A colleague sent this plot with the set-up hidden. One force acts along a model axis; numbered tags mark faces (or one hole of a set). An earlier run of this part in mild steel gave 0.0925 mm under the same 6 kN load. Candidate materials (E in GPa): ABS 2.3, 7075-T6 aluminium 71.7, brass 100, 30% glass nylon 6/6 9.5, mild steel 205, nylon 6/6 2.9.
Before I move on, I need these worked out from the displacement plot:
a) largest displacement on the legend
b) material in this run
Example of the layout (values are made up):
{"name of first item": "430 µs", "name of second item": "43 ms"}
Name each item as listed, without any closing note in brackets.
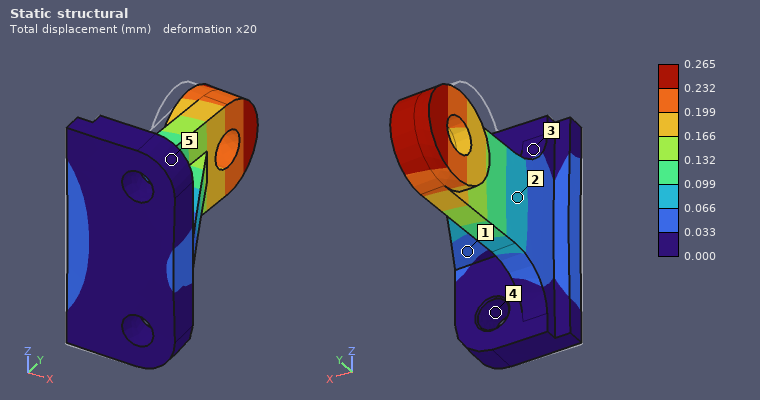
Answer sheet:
{"largest displacement on the legend": "0.265 mm", "material in this run": "7075-T6 aluminium"}
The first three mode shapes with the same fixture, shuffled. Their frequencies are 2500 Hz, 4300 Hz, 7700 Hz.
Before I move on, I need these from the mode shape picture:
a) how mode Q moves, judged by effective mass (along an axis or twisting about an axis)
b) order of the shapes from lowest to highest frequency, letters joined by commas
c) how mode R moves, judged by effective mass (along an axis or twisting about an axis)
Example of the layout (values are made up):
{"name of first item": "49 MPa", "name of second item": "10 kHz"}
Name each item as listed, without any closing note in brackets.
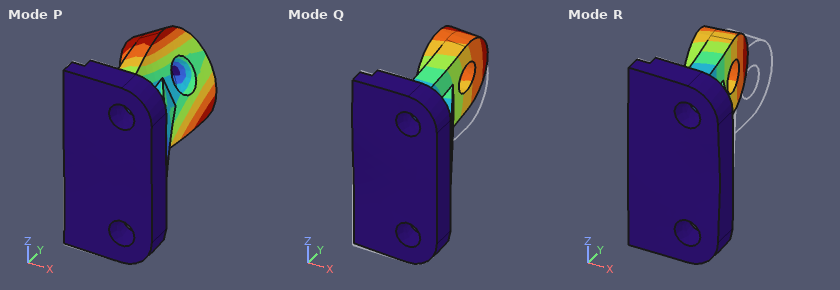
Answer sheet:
{"how mode Q moves, judged by effective mass": "along Z", "order of the shapes from lowest to highest frequency, letters joined by commas": "R, Q, P", "how mode R moves, judged by effective mass": "along X"}
